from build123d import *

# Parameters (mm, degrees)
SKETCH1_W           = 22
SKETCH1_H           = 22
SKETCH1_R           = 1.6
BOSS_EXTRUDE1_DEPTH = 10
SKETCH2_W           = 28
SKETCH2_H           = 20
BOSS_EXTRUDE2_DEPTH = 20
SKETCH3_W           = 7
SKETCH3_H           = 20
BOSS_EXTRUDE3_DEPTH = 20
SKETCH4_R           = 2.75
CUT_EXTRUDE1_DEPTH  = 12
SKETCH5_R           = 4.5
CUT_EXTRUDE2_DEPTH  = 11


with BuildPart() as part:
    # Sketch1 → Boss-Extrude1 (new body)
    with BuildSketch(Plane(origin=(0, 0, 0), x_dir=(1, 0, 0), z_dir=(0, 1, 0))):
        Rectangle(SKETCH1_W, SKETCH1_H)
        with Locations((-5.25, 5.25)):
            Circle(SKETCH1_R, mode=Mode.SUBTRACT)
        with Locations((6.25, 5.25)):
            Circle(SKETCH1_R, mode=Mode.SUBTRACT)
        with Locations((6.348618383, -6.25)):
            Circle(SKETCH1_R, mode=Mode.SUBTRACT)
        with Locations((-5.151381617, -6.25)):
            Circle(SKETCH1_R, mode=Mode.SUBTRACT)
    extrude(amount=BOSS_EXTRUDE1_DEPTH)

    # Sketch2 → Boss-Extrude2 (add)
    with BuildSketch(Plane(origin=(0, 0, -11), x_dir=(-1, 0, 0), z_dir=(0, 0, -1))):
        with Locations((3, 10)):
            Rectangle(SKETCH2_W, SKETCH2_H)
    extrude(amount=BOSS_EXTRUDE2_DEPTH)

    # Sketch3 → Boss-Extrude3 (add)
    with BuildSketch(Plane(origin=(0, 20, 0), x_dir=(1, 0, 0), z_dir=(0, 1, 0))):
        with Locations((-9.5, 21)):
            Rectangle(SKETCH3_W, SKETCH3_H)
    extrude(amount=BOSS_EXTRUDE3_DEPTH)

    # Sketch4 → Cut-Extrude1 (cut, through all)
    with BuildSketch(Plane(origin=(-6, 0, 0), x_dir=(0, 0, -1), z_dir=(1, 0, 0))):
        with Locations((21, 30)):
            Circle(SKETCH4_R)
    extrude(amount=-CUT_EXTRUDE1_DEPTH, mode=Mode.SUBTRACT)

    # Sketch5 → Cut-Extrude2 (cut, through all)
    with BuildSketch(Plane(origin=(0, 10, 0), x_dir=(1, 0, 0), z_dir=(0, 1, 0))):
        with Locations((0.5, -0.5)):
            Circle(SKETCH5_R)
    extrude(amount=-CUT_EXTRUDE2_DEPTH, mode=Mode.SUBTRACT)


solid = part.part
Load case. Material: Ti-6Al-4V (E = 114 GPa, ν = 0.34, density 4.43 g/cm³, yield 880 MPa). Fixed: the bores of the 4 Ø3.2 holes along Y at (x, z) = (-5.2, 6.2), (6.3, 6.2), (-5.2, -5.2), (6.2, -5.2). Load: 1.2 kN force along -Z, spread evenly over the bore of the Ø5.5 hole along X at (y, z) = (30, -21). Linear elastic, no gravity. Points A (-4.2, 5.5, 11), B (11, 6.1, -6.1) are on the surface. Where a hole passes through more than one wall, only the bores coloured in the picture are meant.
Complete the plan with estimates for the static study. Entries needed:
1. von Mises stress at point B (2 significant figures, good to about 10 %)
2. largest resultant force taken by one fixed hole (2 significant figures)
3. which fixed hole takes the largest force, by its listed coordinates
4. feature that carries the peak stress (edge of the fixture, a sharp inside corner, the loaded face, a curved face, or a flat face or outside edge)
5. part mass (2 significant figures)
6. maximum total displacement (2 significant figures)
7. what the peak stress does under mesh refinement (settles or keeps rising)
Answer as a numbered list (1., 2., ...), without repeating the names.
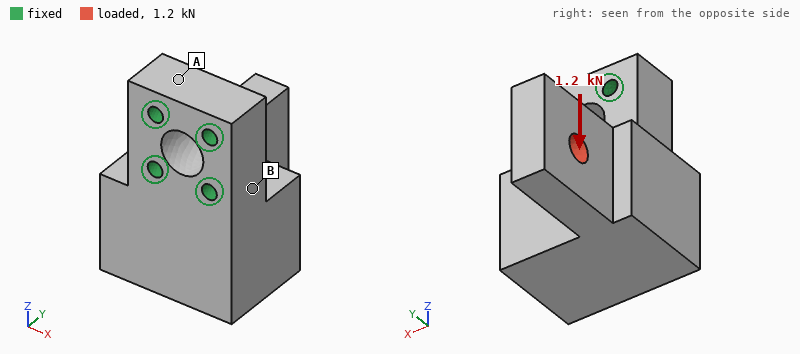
1. 24 MPa
2. 1.3 kN
3. (-5.2, -5.2)
4. edge of the fixture
5. 78 g
6. 77 µm
7. keeps rising
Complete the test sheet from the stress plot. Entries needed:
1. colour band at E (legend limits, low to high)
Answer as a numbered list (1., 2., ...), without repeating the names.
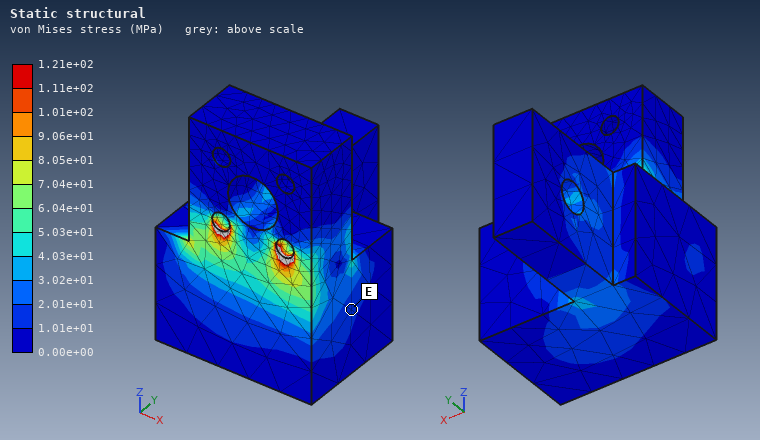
1. 1.01e+01 to 2.01e+01 MPa
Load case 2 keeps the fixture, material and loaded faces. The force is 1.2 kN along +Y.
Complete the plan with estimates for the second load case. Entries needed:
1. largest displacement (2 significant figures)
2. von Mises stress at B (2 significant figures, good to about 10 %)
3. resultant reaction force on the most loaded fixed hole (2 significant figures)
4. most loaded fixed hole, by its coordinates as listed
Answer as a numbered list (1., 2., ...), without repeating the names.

1. 34 µm
2. 19 MPa
3. 1.3 kN
4. (-5.2, -5.2)
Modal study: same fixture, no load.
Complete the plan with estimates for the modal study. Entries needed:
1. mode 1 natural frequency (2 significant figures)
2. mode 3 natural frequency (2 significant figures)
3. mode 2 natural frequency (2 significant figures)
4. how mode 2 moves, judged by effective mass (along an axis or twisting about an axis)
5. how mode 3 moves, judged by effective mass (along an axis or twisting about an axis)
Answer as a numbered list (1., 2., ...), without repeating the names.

1. 4800 Hz
2. 12 kHz
3. 6600 Hz
4. along X
5. along X
